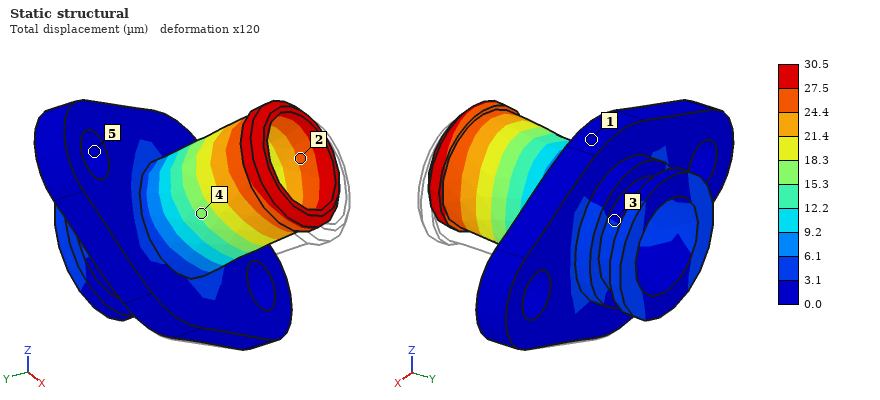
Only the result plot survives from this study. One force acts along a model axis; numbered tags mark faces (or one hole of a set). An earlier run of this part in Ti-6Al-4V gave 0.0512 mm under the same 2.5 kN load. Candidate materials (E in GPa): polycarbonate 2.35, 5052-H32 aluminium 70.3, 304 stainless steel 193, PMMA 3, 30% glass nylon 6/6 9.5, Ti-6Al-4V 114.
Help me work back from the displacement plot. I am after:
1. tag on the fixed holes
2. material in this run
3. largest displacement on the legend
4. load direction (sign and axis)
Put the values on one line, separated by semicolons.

5; 304 stainless steel; 30.5 µm; -X
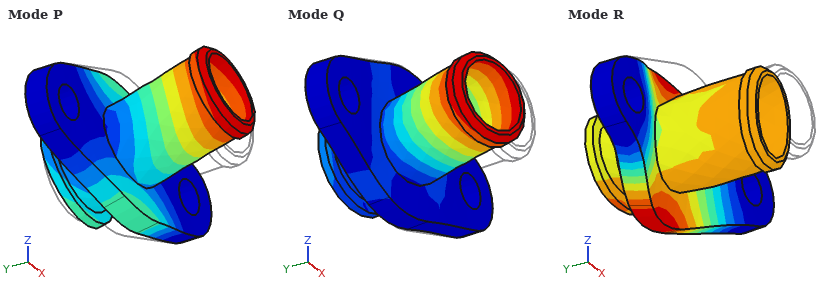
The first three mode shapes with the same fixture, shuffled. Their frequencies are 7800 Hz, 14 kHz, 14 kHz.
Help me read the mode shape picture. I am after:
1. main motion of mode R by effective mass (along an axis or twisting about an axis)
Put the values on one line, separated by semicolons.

along Y
